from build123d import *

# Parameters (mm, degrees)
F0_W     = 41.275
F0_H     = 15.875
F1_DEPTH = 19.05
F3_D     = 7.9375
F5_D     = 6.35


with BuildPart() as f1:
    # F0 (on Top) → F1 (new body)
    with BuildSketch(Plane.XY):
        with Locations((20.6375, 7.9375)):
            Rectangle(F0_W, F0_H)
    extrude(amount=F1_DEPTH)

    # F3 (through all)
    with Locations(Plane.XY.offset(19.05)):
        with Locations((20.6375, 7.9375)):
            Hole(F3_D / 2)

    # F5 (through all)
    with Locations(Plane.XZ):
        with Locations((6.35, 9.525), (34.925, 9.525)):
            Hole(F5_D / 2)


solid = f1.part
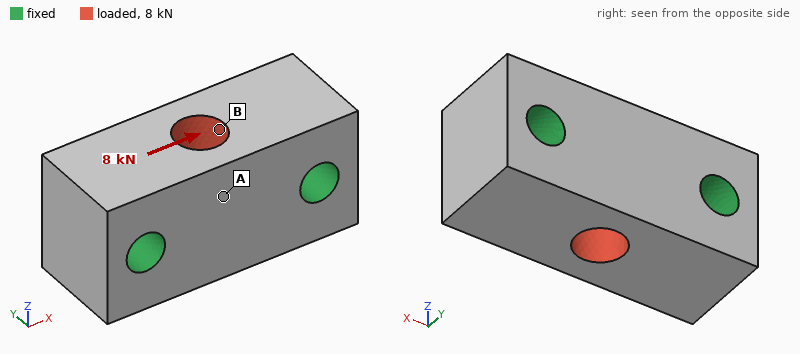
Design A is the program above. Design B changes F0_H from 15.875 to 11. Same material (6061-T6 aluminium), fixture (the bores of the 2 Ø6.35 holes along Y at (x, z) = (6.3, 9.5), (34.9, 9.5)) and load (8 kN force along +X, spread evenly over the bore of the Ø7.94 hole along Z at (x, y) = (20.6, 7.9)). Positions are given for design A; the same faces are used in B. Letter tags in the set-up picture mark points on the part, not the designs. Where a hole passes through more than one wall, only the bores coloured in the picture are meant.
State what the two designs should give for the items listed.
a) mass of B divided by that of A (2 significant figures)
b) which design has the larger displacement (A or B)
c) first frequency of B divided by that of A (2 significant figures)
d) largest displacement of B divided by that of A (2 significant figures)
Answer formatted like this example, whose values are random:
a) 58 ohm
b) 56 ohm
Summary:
a) 0.67
b) B
c) 0.99
d) 1.4
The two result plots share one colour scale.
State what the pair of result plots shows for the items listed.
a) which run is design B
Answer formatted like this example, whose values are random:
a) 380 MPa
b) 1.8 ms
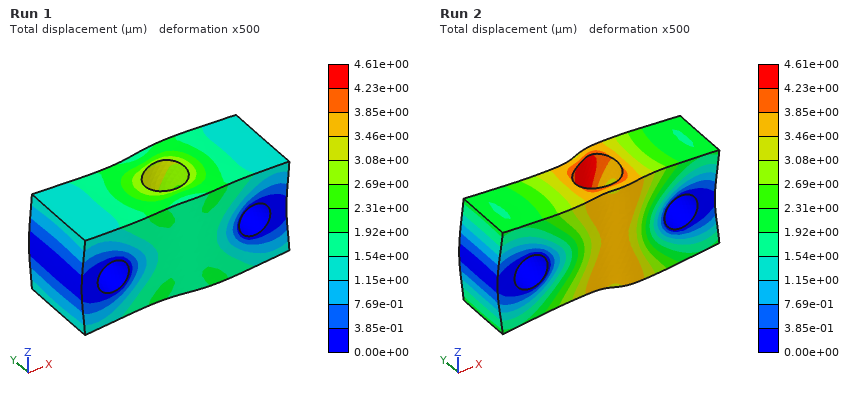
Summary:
a) Run 2
